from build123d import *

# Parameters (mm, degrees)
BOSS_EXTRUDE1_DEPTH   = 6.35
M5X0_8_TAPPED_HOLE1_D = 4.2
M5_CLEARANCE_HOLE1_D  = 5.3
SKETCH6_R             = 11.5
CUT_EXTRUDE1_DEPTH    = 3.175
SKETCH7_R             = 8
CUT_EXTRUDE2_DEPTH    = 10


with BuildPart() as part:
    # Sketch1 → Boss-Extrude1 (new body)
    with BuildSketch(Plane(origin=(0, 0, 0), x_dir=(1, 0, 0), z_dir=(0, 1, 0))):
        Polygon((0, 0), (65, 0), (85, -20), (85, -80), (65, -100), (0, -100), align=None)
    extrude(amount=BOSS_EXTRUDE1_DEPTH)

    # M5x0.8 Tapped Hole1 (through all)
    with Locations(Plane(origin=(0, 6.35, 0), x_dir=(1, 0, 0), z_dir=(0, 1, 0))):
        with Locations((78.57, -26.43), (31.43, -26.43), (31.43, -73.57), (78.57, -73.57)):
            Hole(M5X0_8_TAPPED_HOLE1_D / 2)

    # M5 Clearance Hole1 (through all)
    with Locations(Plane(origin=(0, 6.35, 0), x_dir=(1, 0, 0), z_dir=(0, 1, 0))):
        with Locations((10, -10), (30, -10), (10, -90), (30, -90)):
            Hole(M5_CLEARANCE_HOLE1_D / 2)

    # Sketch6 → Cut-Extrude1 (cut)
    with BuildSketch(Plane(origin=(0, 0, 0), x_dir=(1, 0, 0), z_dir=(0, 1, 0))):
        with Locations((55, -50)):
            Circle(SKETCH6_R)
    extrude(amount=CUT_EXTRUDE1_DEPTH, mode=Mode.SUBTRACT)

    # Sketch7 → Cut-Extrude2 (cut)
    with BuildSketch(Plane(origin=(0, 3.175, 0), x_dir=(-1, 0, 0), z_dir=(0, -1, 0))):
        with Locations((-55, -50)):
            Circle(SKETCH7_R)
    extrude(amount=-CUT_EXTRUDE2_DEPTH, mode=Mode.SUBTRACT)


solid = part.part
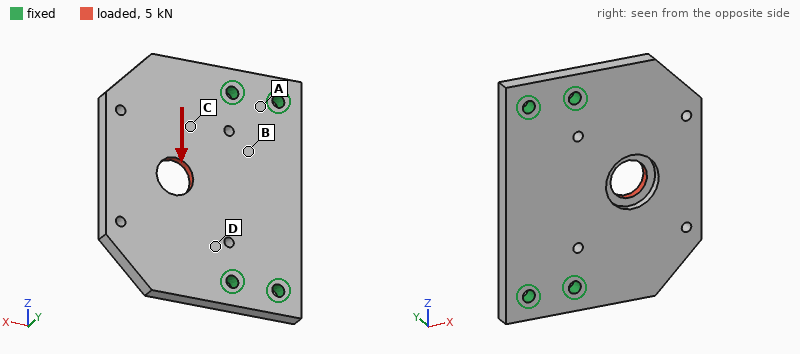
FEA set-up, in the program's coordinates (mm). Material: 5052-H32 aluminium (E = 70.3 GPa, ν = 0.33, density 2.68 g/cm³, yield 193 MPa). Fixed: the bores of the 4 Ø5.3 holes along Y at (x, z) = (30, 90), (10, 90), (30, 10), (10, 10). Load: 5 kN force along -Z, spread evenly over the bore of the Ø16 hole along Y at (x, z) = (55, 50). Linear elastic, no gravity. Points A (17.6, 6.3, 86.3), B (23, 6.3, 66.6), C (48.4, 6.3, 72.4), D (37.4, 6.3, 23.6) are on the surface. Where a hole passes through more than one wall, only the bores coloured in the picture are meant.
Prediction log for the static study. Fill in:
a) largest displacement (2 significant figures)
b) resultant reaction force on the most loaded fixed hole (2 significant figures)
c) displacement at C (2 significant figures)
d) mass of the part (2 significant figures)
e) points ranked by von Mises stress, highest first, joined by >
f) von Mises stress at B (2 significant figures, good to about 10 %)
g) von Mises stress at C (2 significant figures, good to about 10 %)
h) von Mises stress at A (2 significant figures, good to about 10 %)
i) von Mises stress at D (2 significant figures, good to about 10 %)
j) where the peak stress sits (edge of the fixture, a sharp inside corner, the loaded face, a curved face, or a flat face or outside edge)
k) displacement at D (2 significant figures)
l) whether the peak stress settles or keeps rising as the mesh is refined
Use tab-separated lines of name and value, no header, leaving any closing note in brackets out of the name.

largest displacement	23 µm
resultant reaction force on the most loaded fixed hole	2.4 kN
displacement at C	10 µm
mass of the part	130 g
points ranked by von Mises stress, highest first, joined by >	C > D > B > A
von Mises stress at B	8.5 MPa
von Mises stress at C	22 MPa
von Mises stress at A	4.7 MPa
von Mises stress at D	18 MPa
where the peak stress sits	edge of the fixture
displacement at D	5.0 µm
whether the peak stress settles or keeps rising as the mesh is refined	keeps rising
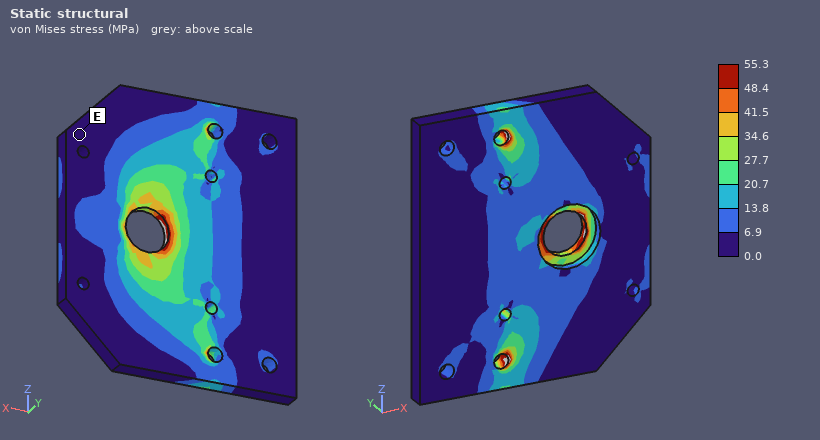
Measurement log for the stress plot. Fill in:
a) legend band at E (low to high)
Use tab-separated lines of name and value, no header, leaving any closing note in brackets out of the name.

legend band at E	0.0 to 6.9 MPa
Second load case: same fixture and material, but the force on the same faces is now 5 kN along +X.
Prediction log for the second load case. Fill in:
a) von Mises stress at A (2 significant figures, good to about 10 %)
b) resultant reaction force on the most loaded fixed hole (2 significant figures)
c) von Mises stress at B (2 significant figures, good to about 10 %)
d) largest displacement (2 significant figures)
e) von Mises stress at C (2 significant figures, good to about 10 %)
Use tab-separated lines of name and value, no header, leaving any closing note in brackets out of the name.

von Mises stress at A	13 MPa
resultant reaction force on the most loaded fixed hole	1.7 kN
von Mises stress at B	14 MPa
largest displacement	80 µm
von Mises stress at C	17 MPa
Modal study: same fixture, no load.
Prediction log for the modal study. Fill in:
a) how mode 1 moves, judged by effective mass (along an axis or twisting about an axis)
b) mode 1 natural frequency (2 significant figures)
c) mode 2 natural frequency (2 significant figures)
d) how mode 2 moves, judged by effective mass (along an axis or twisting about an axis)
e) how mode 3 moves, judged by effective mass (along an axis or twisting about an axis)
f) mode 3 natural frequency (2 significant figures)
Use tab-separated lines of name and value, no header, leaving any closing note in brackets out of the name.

how mode 1 moves, judged by effective mass	along Y
mode 1 natural frequency	1600 Hz
mode 2 natural frequency	3400 Hz
how mode 2 moves, judged by effective mass	twisting about X
how mode 3 moves, judged by effective mass	along Y
mode 3 natural frequency	5100 Hz
